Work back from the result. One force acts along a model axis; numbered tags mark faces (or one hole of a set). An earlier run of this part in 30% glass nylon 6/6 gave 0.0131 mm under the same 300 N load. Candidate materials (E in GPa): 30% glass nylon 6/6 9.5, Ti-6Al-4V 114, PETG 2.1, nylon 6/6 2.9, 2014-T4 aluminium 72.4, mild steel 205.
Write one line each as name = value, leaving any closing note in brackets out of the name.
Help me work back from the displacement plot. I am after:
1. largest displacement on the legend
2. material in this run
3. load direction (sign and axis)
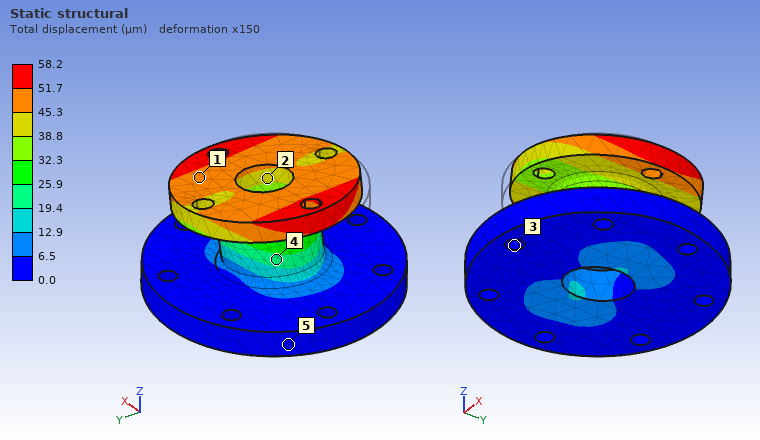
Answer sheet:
largest displacement on the legend = 58.2 µm
material in this run = PETG
load direction = +X
